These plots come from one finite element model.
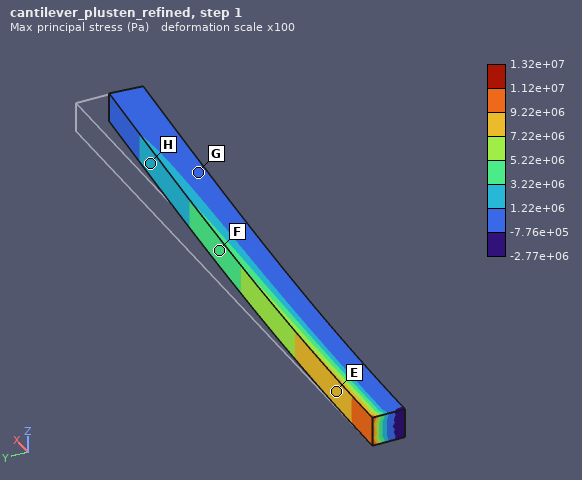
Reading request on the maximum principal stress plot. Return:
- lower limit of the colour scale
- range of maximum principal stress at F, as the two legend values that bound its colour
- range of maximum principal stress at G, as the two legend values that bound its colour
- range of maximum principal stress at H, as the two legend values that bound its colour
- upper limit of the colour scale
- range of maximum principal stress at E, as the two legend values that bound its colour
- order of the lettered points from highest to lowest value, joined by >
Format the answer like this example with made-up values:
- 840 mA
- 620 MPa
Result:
- -2.77e+06 Pa
- 3.22e+06 to 5.22e+06 Pa
- -7.76e+05 to 1.22e+06 Pa
- 1.22e+06 to 3.22e+06 Pa
- 1.32e+07 Pa
- 7.22e+06 to 9.22e+06 Pa
- E > F > H > G
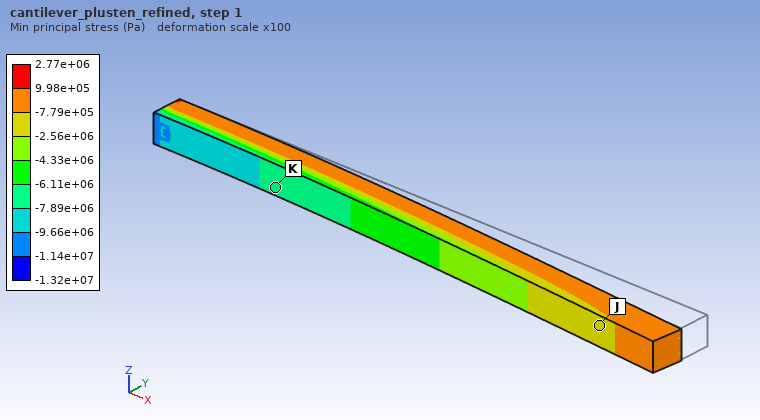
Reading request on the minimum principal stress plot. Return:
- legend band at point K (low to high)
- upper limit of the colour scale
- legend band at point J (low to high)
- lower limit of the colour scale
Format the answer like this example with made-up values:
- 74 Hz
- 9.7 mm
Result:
- -7.89e+06 to -6.11e+06 Pa
- 2.77e+06 Pa
- -2.56e+06 to -7.79e+05 Pa
- -1.32e+07 Pa
